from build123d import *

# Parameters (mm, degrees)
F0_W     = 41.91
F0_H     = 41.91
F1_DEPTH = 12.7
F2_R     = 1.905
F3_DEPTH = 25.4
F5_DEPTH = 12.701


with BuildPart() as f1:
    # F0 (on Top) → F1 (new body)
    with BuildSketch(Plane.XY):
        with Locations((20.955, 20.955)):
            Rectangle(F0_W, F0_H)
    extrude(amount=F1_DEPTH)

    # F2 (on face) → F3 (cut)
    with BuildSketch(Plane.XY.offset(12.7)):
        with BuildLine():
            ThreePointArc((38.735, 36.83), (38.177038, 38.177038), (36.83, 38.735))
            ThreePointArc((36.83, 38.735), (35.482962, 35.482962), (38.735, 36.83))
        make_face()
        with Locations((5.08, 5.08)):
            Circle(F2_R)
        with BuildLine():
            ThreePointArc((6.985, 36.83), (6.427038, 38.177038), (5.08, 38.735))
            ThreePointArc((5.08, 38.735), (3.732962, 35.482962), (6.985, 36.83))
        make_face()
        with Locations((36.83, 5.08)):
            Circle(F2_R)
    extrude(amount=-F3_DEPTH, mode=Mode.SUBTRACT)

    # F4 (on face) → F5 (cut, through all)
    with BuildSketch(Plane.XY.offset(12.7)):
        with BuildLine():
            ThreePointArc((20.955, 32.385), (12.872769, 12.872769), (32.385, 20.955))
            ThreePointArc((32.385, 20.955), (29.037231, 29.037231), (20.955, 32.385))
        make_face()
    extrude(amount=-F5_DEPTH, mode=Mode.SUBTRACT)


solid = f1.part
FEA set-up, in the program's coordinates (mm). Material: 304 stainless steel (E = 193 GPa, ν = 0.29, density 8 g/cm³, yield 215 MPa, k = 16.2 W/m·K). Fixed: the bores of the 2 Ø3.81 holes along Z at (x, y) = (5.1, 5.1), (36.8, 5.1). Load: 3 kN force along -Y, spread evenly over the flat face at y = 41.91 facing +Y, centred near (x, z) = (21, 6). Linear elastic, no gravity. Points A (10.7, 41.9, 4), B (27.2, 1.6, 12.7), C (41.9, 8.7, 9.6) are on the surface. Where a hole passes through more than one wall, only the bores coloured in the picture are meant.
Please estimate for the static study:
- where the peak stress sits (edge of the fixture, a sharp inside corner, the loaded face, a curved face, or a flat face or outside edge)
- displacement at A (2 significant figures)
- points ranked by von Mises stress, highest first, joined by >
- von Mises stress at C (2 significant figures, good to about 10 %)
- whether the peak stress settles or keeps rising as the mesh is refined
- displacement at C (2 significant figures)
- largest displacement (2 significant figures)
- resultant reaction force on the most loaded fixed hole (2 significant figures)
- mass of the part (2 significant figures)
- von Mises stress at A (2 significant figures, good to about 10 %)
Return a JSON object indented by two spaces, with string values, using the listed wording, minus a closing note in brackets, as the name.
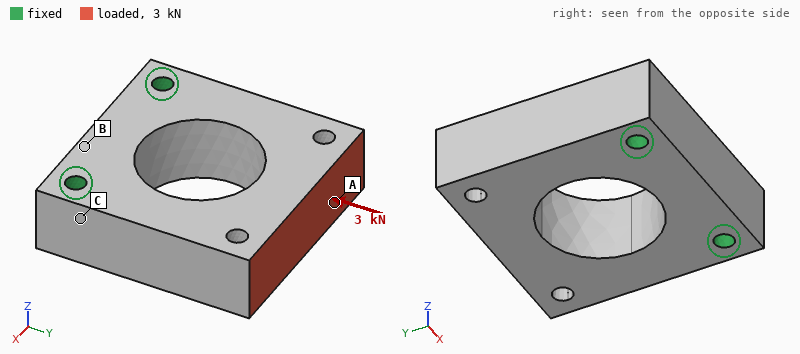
{
  "where the peak stress sits": "edge of the fixture",
  "displacement at A": "2.6 µm",
  "points ranked by von Mises stress, highest first, joined by >": "C > A > B",
  "von Mises stress at C": "11 MPa",
  "whether the peak stress settles or keeps rising as the mesh is refined": "keeps rising",
  "displacement at C": "0.55 µm",
  "largest displacement": "3.4 µm",
  "resultant reaction force on the most loaded fixed hole": "1.5 kN",
  "mass of the part": "130 g",
  "von Mises stress at A": "5.8 MPa"
}
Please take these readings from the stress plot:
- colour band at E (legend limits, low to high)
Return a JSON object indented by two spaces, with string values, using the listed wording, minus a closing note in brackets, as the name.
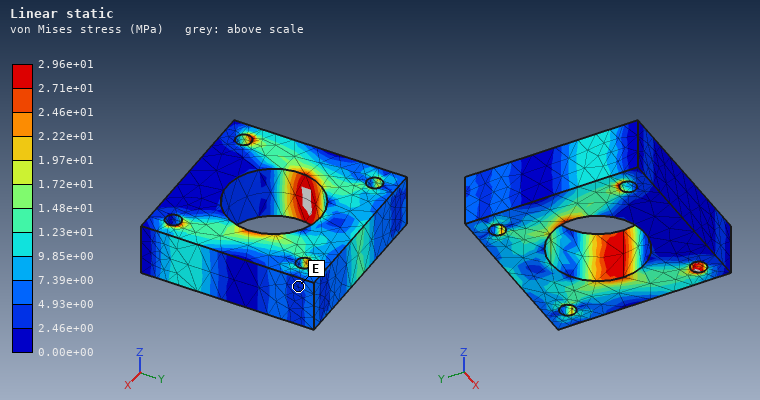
{
  "colour band at E": "2.46e+00 to 4.93e+00 MPa"
}
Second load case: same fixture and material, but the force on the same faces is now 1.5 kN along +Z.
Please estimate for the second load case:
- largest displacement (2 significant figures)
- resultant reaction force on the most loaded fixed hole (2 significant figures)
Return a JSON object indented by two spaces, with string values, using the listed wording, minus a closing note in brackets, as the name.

{
  "largest displacement": "40 µm",
  "resultant reaction force on the most loaded fixed hole": "750 N"
}
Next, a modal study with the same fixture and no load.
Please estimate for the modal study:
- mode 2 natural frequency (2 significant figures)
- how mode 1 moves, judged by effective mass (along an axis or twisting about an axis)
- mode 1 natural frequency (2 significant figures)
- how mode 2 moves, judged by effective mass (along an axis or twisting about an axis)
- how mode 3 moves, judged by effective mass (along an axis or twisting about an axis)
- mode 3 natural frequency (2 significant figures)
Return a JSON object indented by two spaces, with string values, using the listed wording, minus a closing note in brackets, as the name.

{
  "mode 2 natural frequency": "9100 Hz",
  "how mode 1 moves, judged by effective mass": "along Z",
  "mode 1 natural frequency": "5400 Hz",
  "how mode 2 moves, judged by effective mass": "along X",
  "how mode 3 moves, judged by effective mass": "twisting about Y",
  "mode 3 natural frequency": "11 kHz"
}
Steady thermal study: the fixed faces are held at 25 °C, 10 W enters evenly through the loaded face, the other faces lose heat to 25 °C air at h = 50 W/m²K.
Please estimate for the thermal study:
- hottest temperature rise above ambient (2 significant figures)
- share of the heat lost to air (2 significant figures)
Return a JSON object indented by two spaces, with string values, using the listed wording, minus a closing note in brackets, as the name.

{
  "hottest temperature rise above ambient": "48 K",
  "share of the heat lost to air": "51 %"
}
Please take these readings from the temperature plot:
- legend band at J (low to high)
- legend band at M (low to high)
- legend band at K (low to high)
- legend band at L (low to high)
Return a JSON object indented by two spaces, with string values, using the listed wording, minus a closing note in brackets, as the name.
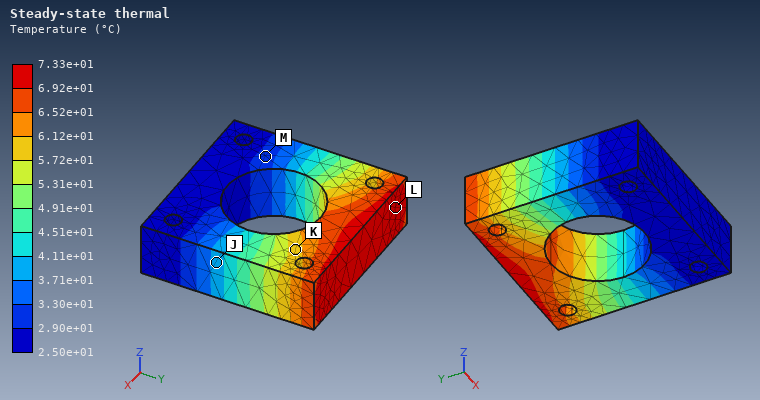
{
  "legend band at J": "3.71e+01 to 4.11e+01 °C",
  "legend band at M": "2.90e+01 to 3.30e+01 °C",
  "legend band at K": "5.72e+01 to 6.12e+01 °C",
  "legend band at L": "6.92e+01 to 7.33e+01 °C"
}
